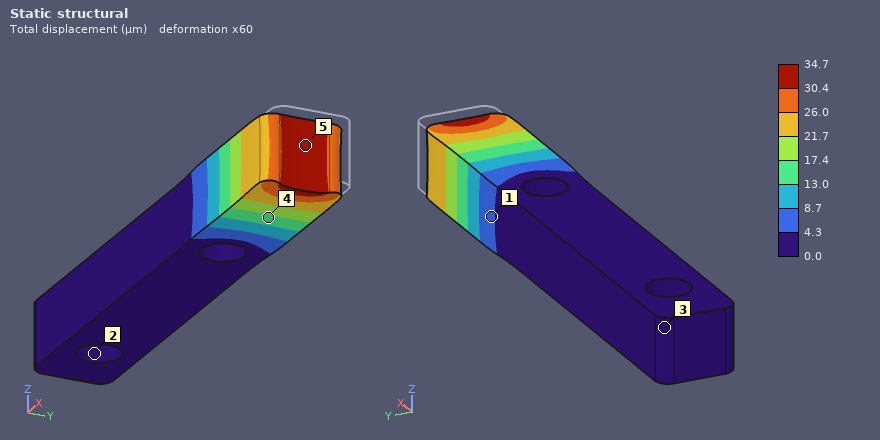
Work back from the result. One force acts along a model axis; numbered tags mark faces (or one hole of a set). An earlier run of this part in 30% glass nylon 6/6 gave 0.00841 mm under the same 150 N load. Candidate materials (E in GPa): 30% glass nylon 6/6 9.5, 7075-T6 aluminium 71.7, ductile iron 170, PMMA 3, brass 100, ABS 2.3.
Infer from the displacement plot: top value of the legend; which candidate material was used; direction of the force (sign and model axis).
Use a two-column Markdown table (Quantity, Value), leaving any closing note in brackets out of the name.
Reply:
| Quantity | Value |
|---|---|
| top value of the legend | 34.7 µm |
| which candidate material was used | ABS |
| direction of the force | -X |
